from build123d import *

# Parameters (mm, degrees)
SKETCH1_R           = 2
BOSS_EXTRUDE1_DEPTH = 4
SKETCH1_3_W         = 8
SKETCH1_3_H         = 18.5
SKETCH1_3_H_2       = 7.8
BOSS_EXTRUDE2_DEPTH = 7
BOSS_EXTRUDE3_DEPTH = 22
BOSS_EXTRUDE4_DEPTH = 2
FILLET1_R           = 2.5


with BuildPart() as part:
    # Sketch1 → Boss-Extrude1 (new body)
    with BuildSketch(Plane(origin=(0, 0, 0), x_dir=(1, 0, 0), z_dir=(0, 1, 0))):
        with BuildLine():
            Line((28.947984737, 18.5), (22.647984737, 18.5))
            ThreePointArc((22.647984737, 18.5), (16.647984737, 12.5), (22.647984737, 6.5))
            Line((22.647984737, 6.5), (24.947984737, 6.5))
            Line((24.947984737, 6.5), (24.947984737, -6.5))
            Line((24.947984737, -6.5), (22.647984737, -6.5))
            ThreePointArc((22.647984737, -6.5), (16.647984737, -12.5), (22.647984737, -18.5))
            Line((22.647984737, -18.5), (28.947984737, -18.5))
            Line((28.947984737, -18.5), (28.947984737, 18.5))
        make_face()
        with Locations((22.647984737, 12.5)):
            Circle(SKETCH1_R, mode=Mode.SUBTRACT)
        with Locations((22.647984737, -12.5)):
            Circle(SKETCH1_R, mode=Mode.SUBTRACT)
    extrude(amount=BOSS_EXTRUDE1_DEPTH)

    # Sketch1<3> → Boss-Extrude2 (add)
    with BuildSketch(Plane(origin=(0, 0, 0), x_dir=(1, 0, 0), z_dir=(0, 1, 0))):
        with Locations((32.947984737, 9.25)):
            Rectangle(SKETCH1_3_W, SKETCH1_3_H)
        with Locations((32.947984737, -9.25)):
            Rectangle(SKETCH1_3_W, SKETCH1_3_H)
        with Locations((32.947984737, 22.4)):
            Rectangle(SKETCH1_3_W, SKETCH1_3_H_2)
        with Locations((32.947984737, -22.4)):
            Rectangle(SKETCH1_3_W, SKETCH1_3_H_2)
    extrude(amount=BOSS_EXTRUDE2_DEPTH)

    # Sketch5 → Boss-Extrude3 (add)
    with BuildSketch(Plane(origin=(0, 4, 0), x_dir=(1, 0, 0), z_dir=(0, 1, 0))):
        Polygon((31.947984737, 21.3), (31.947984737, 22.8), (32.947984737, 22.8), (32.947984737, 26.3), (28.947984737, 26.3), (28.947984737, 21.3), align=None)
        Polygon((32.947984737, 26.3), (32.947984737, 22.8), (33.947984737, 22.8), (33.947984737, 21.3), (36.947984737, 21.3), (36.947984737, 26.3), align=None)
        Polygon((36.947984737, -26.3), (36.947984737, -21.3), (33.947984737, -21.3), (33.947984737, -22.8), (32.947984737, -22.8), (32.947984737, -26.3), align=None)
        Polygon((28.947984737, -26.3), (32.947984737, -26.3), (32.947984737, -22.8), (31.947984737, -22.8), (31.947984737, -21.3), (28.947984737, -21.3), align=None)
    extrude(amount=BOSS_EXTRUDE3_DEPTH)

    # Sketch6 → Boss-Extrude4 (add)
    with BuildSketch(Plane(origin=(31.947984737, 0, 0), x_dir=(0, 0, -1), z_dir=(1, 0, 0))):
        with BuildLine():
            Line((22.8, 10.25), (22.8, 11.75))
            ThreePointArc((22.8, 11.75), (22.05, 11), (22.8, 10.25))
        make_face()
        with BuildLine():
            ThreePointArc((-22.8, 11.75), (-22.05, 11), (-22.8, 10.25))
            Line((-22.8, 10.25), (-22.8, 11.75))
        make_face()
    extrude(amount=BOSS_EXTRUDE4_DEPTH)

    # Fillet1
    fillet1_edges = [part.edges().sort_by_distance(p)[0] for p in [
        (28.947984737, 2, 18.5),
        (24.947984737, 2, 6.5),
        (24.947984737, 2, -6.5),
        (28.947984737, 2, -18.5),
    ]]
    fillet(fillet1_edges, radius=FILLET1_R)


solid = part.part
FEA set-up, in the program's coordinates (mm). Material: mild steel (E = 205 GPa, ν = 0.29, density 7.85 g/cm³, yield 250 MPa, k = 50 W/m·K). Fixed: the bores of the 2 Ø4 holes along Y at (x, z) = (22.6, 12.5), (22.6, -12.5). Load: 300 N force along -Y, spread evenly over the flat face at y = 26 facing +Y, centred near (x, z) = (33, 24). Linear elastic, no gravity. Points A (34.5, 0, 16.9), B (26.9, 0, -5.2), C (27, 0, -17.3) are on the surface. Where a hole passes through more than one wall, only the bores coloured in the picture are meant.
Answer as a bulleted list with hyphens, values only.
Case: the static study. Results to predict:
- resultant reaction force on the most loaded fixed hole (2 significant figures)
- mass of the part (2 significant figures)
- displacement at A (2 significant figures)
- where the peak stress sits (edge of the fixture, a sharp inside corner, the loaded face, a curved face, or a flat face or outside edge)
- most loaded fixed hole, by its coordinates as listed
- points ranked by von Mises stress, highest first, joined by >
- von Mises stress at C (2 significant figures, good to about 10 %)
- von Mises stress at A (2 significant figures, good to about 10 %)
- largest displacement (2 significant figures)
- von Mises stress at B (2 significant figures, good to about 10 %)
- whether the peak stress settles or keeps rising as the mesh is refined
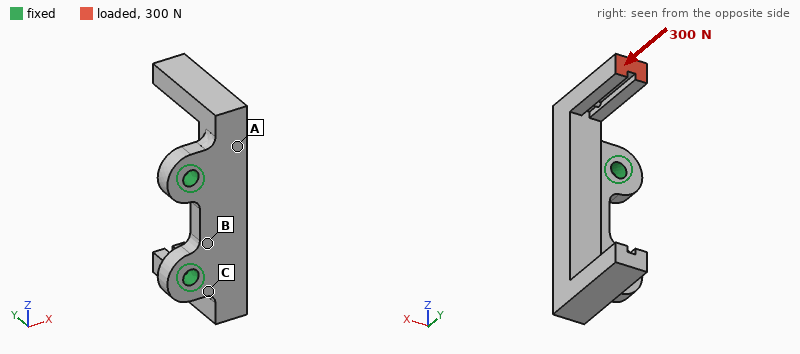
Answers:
- 380 N
- 43 g
- 9.6 µm
- edge of the fixture
- (22.6, 12.5)
- A > B > C
- 7.9 MPa
- 27 MPa
- 34 µm
- 17 MPa
- keeps rising
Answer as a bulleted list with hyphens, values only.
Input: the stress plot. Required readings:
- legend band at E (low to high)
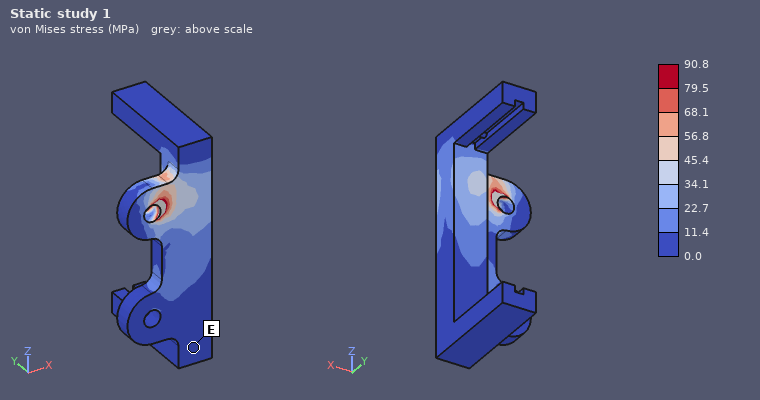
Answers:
- 0.0 to 11.4 MPa
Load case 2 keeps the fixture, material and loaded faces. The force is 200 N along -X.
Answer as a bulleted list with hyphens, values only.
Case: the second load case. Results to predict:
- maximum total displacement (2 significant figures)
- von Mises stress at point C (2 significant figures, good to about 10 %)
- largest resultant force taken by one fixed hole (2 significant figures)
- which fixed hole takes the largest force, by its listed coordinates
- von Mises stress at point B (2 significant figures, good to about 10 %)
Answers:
- 85 µm
- 33 MPa
- 290 N
- (22.6, 12.5)
- 40 MPa
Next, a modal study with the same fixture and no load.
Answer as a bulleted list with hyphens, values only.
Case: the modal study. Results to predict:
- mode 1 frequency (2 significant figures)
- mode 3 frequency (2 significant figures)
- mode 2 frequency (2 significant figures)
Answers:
- 4300 Hz
- 5600 Hz
- 4800 Hz
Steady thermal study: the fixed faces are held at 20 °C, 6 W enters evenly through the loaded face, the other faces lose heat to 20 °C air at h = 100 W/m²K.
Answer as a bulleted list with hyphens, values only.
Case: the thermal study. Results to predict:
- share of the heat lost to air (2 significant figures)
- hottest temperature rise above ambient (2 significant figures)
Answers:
- 53 %
- 68 K
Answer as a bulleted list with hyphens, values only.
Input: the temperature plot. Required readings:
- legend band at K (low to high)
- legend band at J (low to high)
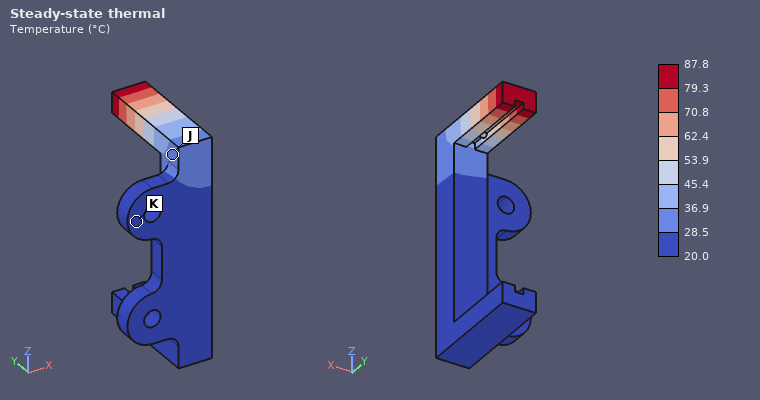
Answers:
- 20.0 to 28.5 °C
- 28.5 to 36.9 °C
